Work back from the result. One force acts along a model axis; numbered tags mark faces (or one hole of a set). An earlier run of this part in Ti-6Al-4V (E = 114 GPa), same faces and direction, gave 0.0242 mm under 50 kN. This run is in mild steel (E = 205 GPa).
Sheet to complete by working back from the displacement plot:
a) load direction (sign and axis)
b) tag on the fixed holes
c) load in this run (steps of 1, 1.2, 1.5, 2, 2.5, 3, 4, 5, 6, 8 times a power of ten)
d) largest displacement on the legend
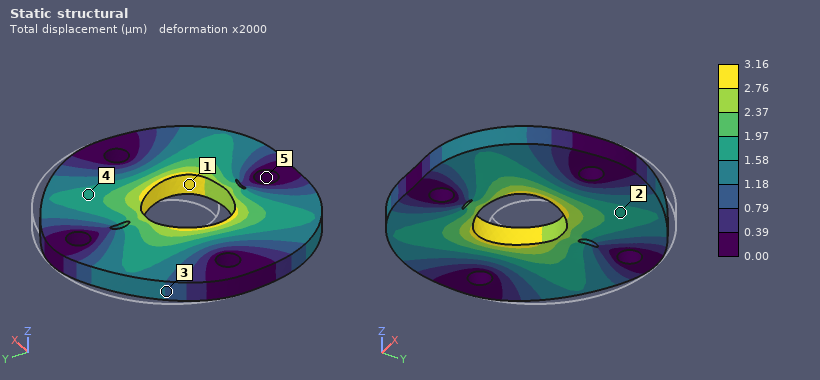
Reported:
-Y
5
12 kN
3.16 µm
